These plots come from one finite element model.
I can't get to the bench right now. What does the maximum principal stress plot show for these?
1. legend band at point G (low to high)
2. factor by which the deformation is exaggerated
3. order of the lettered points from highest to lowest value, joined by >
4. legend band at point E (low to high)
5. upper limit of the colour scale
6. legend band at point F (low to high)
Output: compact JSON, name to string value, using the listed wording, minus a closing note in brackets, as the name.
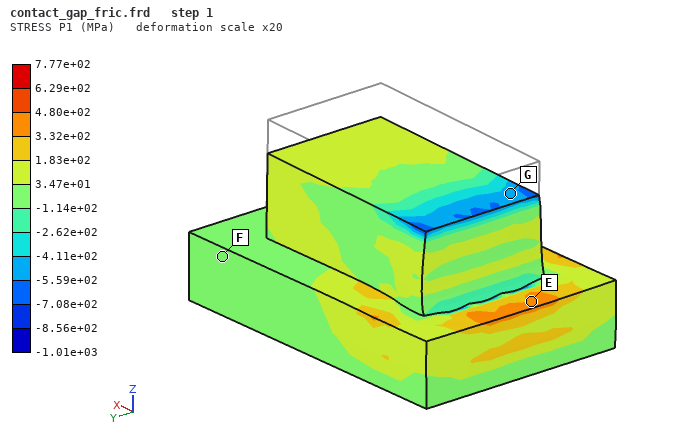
{"legend band at point G": "-5.59e+02 to -4.11e+02 MPa", "factor by which the deformation is exaggerated": "20", "order of the lettered points from highest to lowest value, joined by >": "E > F > G", "legend band at point E": "3.32e+02 to 4.80e+02 MPa", "upper limit of the colour scale": "7.77e+02 MPa", "legend band at point F": "-1.14e+02 to 3.47e+01 MPa"}
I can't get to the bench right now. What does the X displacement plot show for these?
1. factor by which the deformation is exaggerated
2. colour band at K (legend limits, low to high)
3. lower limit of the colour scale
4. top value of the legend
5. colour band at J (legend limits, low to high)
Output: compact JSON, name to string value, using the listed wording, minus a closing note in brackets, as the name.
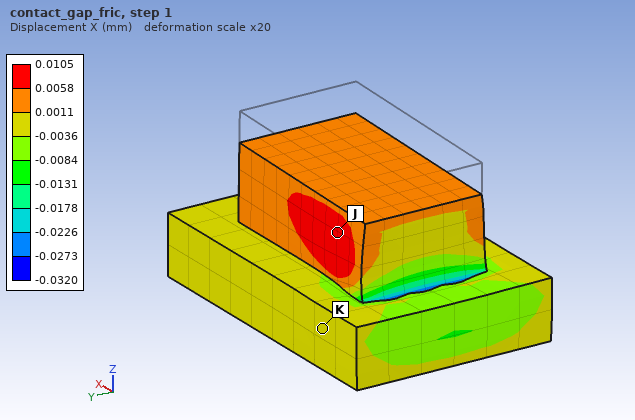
{"factor by which the deformation is exaggerated": "20", "colour band at K": "-0.0036 to 0.0011 mm", "lower limit of the colour scale": "-0.0320 mm", "top value of the legend": "0.0105 mm", "colour band at J": "0.0058 to 0.0105 mm"}
